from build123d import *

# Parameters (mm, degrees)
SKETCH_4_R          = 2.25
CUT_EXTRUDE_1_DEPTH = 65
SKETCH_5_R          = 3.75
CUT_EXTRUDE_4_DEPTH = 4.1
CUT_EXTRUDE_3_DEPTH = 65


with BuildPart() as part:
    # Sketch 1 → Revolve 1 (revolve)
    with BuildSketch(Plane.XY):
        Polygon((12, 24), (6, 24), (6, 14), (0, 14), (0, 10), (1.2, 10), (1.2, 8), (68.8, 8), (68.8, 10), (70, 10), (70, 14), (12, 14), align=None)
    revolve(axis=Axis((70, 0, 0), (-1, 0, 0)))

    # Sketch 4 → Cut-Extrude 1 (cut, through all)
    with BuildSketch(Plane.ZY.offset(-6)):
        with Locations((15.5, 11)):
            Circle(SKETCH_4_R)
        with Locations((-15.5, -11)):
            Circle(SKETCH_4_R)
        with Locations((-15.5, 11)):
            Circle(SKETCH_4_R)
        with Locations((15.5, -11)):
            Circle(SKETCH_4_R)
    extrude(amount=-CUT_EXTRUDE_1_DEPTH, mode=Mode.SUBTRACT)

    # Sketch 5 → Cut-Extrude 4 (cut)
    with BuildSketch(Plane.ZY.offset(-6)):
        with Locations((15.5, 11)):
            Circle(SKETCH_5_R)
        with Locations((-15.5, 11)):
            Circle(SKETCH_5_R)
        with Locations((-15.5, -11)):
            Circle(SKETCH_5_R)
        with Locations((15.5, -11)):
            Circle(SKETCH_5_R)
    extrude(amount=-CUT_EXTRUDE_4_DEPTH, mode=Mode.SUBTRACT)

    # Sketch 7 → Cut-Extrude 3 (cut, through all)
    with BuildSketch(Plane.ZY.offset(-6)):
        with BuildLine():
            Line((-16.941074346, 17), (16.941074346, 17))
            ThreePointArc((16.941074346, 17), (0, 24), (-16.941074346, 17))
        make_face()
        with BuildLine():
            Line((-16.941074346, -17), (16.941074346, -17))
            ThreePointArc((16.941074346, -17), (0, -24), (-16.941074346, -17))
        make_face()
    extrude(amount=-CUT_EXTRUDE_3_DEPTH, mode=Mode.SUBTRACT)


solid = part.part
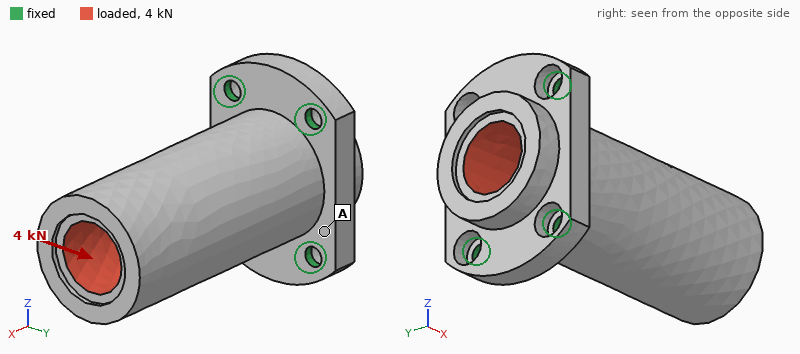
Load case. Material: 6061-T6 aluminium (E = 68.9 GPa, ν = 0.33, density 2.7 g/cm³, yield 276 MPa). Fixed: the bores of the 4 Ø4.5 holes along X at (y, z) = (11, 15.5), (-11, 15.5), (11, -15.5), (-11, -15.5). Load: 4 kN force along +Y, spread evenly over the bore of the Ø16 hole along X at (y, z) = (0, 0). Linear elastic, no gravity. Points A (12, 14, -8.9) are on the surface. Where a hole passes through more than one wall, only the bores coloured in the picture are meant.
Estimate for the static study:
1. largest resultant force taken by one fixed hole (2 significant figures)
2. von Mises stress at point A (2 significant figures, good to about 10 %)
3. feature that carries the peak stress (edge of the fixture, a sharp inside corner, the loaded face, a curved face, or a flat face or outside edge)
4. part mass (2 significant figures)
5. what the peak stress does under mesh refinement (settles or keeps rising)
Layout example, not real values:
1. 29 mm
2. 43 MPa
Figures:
1. 2.4 kN
2. 58 MPa
3. edge of the fixture
4. 89 g
5. keeps rising
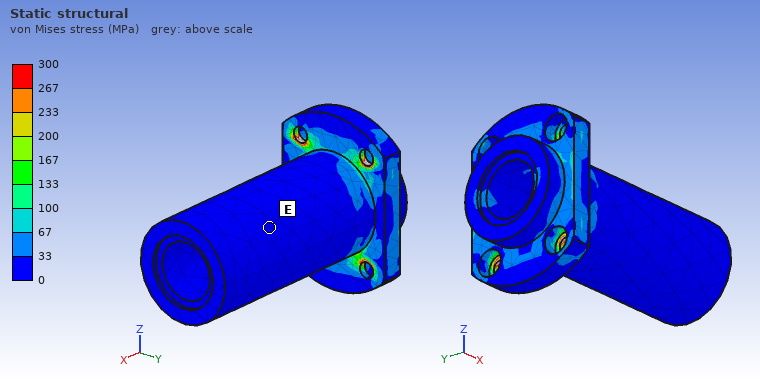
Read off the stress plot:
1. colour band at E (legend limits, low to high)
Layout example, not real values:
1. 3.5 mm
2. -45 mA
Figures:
1. 0 to 33 MPa
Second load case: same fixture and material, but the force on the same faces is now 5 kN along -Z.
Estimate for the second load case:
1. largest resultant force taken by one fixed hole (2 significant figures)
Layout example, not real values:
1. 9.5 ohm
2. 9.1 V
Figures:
1. 2.4 kN
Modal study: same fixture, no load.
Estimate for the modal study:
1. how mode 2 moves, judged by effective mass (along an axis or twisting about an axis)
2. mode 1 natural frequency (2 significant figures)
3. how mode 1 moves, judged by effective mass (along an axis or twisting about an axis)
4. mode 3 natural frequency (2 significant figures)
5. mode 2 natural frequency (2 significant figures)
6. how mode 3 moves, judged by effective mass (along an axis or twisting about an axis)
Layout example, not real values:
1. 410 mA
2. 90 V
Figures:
1. along Z
2. 3000 Hz
3. along Y
4. 10 kHz
5. 3800 Hz
6. along X
